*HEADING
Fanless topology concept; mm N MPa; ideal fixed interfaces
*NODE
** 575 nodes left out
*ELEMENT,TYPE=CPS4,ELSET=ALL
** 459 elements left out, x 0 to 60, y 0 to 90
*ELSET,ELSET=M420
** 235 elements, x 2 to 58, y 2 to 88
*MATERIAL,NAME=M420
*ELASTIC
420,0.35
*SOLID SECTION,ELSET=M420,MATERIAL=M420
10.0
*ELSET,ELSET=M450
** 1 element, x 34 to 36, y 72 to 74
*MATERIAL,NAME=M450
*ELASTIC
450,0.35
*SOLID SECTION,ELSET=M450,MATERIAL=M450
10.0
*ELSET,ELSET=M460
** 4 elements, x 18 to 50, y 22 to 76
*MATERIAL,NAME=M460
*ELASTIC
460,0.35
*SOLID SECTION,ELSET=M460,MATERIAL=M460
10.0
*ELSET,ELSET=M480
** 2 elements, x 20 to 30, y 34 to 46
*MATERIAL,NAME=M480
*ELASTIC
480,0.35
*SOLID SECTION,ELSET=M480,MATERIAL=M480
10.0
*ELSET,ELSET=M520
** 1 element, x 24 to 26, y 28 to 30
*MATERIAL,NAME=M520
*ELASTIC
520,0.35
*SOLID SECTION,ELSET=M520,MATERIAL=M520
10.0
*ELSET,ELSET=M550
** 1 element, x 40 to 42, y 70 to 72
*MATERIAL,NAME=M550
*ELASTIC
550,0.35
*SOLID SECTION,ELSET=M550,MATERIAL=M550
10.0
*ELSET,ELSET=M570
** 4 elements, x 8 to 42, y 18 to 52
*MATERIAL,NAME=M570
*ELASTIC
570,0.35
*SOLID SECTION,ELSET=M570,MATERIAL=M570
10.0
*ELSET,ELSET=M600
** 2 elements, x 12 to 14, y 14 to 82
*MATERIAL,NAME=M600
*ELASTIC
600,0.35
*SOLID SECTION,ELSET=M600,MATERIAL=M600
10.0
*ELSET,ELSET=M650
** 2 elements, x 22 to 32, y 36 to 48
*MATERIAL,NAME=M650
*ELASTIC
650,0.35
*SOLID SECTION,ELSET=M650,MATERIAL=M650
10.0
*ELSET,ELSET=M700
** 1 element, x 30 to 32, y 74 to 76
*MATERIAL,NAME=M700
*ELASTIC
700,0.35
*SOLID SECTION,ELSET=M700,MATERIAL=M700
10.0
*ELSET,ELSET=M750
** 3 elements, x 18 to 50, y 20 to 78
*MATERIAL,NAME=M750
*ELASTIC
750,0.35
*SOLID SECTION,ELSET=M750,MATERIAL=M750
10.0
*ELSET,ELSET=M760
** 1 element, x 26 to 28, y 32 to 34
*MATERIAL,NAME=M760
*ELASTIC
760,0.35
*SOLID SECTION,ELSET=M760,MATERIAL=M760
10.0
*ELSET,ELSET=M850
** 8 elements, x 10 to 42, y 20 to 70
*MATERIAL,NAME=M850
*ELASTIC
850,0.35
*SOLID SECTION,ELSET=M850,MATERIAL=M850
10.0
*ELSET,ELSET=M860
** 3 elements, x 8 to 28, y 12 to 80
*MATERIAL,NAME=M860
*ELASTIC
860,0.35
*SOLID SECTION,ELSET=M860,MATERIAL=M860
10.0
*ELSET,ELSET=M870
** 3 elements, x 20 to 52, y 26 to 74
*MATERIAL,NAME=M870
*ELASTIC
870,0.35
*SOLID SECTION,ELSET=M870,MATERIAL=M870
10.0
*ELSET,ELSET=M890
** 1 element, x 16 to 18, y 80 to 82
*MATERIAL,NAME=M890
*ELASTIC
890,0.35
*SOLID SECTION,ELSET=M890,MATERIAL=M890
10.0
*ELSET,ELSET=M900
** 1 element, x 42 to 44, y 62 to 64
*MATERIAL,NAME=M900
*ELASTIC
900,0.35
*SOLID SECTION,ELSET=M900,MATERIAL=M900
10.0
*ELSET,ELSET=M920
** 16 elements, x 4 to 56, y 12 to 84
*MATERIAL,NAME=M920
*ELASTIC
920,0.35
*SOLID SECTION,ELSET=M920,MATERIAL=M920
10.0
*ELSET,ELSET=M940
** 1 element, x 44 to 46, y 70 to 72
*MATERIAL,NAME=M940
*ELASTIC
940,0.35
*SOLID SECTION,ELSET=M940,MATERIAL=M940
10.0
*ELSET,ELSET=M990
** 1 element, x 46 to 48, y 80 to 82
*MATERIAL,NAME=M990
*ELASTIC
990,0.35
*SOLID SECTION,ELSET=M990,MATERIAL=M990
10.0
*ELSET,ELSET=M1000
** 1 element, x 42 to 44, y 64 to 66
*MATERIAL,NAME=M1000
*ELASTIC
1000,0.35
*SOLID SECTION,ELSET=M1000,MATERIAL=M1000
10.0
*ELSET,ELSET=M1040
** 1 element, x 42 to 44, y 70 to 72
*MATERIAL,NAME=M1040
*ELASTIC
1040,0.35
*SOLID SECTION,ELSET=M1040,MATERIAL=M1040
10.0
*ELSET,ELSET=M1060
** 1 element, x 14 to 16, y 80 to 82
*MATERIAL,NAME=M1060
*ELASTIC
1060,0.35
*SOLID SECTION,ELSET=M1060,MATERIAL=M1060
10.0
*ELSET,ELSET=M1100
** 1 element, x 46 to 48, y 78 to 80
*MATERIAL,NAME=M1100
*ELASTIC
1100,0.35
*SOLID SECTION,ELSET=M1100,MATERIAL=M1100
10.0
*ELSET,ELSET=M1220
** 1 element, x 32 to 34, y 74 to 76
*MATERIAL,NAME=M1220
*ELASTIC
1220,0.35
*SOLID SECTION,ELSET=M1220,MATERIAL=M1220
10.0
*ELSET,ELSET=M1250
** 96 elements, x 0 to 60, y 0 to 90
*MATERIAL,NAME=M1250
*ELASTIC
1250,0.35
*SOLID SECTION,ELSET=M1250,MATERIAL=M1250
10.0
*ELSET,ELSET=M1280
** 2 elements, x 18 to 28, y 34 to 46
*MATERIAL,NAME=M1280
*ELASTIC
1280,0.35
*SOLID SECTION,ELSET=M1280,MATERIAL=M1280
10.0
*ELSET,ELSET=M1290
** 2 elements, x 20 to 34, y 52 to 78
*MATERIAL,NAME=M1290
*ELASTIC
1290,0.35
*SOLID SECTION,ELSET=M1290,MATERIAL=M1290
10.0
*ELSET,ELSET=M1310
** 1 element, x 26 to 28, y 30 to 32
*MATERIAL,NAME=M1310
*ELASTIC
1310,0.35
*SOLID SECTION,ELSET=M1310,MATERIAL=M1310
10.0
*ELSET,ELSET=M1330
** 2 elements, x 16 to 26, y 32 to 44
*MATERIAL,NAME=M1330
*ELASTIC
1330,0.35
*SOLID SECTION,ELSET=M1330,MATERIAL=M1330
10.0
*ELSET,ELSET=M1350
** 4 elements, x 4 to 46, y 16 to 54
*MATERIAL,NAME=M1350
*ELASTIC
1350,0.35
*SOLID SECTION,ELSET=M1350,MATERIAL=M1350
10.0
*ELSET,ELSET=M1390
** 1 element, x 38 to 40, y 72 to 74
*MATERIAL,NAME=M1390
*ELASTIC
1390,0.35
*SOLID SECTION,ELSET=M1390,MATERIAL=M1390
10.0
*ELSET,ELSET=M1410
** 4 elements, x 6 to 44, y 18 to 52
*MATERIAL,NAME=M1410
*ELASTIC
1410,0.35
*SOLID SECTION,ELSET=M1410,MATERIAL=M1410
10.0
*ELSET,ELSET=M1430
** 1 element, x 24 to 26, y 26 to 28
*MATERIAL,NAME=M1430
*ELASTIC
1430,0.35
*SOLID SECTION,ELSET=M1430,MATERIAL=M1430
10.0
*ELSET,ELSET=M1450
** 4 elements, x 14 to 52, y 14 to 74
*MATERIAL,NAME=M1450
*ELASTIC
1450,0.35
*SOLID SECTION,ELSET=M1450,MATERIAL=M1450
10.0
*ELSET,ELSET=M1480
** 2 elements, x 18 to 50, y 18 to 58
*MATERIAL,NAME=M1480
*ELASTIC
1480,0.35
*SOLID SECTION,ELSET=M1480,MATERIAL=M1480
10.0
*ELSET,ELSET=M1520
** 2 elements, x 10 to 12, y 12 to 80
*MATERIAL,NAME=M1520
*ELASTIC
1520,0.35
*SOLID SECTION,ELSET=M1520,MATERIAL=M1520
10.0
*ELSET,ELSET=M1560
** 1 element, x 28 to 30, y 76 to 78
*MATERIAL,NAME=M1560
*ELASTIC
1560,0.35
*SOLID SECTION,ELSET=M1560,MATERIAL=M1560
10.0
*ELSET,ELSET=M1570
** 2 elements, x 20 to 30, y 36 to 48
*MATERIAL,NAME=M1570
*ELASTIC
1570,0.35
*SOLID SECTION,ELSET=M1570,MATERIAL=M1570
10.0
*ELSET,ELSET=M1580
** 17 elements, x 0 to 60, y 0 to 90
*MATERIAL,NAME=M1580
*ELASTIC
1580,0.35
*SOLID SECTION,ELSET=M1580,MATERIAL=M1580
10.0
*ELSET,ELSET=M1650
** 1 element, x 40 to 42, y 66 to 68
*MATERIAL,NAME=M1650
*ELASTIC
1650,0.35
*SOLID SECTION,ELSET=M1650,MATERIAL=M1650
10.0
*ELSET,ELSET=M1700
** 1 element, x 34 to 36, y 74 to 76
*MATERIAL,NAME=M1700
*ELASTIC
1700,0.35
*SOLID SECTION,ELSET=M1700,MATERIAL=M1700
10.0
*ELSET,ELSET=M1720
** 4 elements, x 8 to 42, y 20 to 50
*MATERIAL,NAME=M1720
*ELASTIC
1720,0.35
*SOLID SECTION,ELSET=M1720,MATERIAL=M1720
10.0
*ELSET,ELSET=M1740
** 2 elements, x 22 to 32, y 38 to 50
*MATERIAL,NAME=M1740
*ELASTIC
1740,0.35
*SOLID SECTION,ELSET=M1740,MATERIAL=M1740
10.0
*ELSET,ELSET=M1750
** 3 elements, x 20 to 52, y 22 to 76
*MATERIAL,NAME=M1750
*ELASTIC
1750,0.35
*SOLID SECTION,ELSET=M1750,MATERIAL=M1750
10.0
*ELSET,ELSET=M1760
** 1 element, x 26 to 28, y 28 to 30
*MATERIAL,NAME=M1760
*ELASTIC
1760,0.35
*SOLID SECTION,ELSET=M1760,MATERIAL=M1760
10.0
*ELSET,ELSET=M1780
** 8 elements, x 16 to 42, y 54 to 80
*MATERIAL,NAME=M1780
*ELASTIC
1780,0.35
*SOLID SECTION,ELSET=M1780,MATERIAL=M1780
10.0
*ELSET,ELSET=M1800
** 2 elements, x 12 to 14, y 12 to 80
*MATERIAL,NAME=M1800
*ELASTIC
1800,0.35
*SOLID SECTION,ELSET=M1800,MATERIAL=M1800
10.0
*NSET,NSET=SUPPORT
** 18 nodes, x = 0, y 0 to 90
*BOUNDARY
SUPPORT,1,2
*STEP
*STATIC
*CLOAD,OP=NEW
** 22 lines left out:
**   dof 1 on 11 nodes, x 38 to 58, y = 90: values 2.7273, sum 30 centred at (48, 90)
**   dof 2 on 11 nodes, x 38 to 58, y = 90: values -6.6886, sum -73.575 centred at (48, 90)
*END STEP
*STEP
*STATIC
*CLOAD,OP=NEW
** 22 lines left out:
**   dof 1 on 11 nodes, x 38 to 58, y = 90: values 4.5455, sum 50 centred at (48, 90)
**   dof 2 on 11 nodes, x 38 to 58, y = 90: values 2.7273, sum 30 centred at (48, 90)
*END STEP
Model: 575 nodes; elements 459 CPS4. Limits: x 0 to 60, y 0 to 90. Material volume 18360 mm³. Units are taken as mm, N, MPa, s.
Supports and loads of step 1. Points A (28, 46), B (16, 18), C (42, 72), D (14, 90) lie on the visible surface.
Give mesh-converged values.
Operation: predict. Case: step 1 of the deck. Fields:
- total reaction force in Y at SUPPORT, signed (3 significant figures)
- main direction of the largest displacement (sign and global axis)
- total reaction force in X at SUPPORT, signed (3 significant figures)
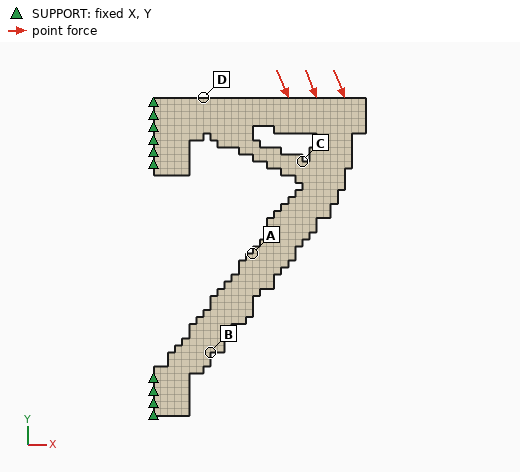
73.6 N
-Y
-30.0 N
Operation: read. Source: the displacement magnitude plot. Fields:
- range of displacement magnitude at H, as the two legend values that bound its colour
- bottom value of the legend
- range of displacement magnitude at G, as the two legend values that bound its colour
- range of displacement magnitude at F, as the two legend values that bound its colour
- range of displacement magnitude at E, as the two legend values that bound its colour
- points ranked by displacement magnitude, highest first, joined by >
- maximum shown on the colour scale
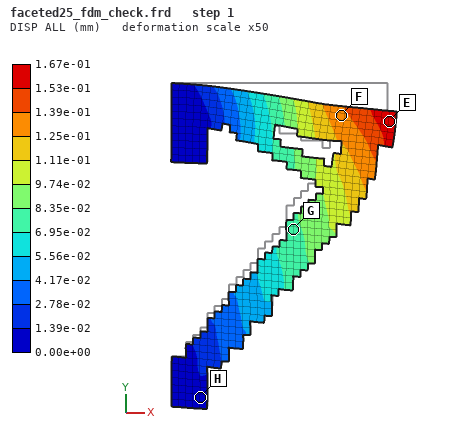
0.00e+00 to 1.39e-02 mm
0.00e+00 mm
6.95e-02 to 8.35e-02 mm
1.25e-01 to 1.39e-01 mm
1.53e-01 to 1.67e-01 mm
E > F > G > H
1.67e-01 mm
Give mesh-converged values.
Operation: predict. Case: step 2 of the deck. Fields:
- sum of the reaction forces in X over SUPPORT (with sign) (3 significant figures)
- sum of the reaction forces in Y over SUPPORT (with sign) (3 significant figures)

-50.0 N
-30.0 N
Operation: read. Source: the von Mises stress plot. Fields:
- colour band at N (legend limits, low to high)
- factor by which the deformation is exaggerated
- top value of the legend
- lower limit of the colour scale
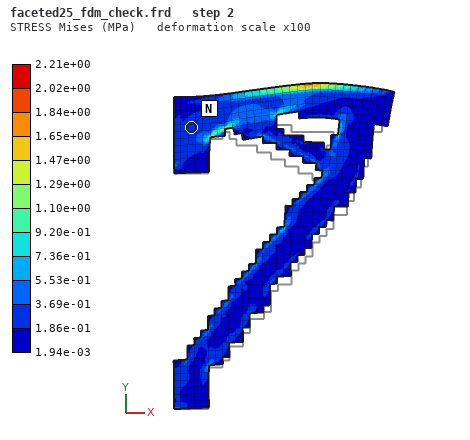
1.86e-01 to 3.69e-01 MPa
100
2.21e+00 MPa
1.94e-03 MPa
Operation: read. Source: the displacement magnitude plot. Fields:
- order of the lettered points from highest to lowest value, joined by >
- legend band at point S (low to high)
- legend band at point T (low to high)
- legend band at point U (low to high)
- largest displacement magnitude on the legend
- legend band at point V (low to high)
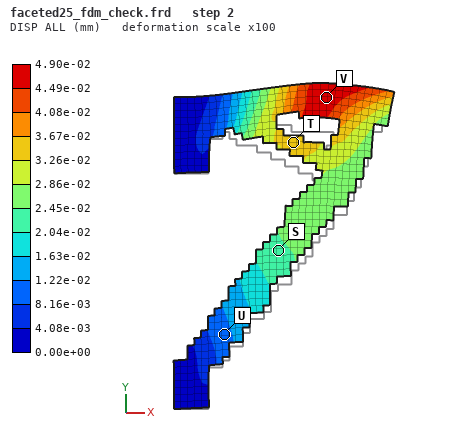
V > T > S > U
2.04e-02 to 2.45e-02 mm
3.26e-02 to 3.67e-02 mm
8.16e-03 to 1.22e-02 mm
4.90e-02 mm
4.49e-02 to 4.90e-02 mm
